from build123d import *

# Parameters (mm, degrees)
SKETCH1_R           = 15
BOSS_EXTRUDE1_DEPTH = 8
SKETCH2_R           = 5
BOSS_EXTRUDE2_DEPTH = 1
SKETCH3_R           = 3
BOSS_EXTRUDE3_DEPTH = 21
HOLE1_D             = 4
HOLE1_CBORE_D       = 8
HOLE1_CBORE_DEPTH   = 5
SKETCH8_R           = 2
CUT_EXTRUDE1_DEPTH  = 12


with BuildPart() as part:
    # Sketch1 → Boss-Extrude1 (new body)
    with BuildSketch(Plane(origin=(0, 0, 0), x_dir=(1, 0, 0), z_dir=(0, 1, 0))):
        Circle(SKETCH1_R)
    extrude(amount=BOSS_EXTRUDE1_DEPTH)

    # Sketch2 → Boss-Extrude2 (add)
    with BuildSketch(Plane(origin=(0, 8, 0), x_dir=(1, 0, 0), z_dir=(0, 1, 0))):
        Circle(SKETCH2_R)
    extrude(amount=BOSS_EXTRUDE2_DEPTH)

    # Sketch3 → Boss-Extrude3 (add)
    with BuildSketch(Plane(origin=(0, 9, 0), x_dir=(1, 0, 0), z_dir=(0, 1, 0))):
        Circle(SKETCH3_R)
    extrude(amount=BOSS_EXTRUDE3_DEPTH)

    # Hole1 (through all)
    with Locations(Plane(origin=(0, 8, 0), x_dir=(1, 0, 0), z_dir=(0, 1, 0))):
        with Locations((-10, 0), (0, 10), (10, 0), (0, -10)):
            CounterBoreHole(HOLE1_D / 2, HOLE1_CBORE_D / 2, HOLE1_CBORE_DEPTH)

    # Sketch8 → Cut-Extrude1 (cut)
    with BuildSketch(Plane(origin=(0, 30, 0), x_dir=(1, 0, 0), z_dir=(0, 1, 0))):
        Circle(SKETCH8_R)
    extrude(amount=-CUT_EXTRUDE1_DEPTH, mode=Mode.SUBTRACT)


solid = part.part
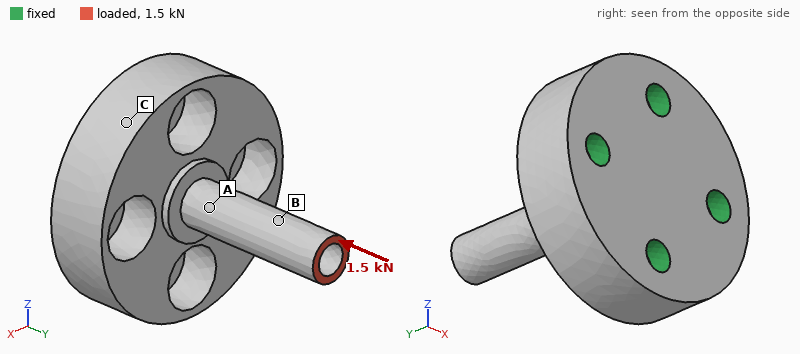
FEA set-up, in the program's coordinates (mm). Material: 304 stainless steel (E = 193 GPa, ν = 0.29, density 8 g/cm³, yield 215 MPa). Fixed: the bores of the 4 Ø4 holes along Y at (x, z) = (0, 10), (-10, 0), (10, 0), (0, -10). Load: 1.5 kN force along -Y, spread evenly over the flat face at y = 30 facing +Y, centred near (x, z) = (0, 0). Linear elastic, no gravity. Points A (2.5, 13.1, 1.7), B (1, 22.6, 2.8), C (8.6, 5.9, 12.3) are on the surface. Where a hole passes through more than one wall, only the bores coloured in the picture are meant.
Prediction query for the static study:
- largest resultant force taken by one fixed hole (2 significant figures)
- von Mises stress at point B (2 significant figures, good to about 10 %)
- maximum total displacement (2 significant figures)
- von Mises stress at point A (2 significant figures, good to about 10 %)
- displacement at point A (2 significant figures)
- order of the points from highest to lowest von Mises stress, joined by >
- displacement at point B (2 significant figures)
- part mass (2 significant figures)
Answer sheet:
410 N
96 MPa
10 µm
53 MPa
2.7 µm
B > A > C
6.6 µm
40 g
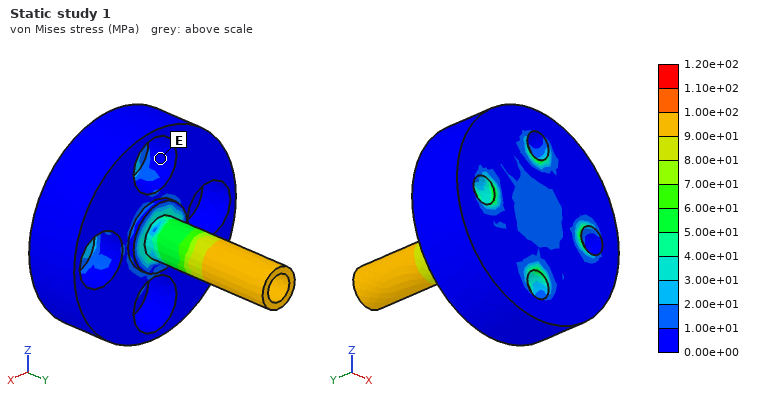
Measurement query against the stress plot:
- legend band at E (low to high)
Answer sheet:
0.00e+00 to 1.00e+01 MPa
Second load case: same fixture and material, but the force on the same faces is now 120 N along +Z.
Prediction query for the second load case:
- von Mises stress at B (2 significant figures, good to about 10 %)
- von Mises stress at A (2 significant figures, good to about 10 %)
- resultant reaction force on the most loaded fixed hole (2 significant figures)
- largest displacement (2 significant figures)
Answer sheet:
49 MPa
55 MPa
170 N
43 µm
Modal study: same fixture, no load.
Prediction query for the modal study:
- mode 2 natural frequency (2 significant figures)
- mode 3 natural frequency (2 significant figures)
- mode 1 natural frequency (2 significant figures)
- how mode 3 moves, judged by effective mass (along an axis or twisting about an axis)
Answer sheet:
10 kHz
37 kHz
10 kHz
along X
